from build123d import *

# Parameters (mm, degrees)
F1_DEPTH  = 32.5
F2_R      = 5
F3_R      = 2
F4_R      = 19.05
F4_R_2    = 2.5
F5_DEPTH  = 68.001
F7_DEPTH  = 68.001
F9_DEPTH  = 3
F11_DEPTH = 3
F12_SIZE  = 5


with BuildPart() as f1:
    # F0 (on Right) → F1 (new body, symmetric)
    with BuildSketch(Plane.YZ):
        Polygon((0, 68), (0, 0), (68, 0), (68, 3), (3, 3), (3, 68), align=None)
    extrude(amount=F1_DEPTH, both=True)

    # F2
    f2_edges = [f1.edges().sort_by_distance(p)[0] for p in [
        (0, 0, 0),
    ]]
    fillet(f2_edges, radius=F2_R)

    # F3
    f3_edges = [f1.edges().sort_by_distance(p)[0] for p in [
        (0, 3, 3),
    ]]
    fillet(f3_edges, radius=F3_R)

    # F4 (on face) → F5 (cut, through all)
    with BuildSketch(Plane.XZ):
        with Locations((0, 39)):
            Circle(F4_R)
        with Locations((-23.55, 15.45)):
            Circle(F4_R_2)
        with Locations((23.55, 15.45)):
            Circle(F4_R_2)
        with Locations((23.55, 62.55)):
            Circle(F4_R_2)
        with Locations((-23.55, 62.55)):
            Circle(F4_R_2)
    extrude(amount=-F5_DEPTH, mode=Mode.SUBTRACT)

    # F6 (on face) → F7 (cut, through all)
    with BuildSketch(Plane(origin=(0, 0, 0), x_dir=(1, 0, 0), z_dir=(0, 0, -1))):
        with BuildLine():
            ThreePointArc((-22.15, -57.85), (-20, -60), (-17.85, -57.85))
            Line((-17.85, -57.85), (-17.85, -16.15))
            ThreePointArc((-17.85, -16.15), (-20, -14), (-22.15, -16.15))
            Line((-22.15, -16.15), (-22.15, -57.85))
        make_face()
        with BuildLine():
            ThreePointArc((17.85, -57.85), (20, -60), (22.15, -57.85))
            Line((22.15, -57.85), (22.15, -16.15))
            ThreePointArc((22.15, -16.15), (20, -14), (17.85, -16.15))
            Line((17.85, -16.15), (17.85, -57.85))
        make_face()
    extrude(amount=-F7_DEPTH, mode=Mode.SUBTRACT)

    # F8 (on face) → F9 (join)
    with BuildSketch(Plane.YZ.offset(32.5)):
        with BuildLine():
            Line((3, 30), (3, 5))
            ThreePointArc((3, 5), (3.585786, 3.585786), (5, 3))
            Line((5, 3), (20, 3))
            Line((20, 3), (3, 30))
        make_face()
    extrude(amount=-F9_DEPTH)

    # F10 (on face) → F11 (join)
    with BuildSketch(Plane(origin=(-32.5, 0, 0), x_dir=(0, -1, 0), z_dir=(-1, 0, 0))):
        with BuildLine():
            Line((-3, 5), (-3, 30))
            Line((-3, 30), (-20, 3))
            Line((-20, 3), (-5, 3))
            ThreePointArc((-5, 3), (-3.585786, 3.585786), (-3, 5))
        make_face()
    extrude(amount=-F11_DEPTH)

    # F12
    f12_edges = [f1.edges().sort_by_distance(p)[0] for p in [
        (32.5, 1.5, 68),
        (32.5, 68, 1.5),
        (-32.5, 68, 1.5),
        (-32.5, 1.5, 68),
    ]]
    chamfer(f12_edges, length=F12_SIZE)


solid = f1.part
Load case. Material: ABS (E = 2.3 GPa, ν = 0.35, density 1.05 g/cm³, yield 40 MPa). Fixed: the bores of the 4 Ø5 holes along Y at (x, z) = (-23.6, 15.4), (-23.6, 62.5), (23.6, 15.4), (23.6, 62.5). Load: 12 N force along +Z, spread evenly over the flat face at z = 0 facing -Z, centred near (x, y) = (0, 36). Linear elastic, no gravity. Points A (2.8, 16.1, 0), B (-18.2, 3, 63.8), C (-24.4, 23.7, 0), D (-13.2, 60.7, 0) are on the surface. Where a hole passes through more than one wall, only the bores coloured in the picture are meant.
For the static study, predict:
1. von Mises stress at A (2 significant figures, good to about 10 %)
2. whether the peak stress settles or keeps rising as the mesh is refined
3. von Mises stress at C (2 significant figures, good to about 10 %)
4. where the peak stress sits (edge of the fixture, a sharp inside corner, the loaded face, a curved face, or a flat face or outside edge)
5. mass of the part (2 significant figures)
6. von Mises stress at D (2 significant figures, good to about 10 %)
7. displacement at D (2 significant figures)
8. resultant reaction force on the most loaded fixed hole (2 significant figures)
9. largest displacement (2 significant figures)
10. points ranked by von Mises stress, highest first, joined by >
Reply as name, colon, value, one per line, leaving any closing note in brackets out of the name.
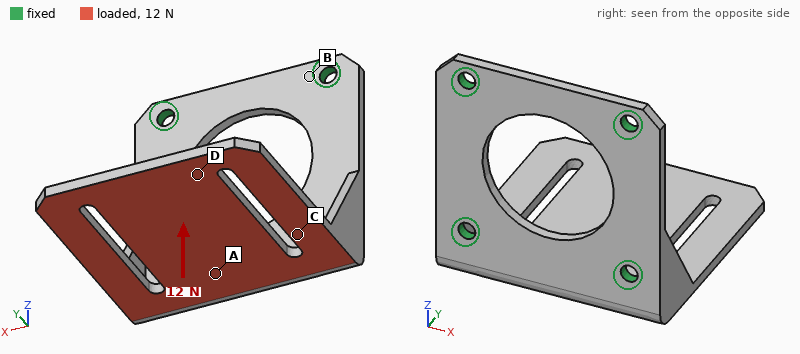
von Mises stress at A: 1.6 MPa
whether the peak stress settles or keeps rising as the mesh is refined: keeps rising
von Mises stress at C: 3.3 MPa
where the peak stress sits: edge of the fixture
mass of the part: 23 g
von Mises stress at D: 0.80 MPa
displacement at D: 1.1 mm
resultant reaction force on the most loaded fixed hole: 6.6 N
largest displacement: 1.3 mm
points ranked by von Mises stress, highest first, joined by >: C > A > D > B
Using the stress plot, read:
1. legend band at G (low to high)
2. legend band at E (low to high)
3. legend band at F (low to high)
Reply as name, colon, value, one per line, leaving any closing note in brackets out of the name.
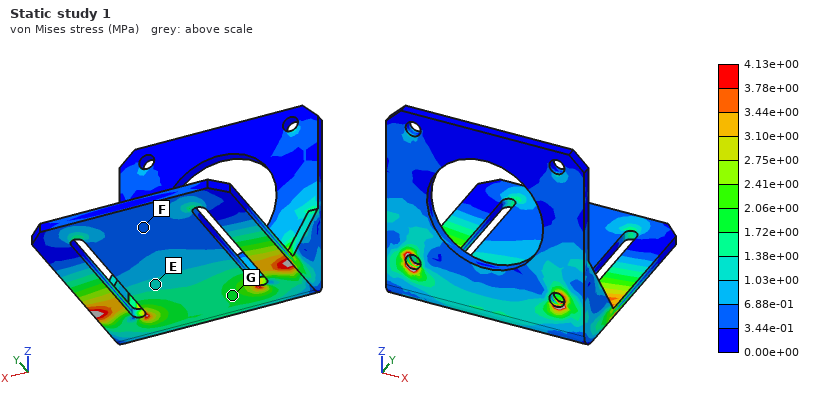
legend band at G: 1.72e+00 to 2.06e+00 MPa
legend band at E: 1.03e+00 to 1.38e+00 MPa
legend band at F: 3.44e-01 to 6.88e-01 MPa
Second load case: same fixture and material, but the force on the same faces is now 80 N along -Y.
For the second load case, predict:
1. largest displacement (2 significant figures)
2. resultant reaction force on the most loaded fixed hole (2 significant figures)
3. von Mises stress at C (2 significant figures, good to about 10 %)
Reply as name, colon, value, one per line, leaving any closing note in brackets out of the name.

largest displacement: 1.2 mm
resultant reaction force on the most loaded fixed hole: 44 N
von Mises stress at C: 1.7 MPa
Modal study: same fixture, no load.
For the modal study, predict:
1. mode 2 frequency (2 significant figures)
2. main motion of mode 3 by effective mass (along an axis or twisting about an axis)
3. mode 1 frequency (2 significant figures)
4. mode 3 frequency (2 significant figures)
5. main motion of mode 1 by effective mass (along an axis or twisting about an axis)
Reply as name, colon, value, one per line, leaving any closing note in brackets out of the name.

mode 2 frequency: 450 Hz
main motion of mode 3 by effective mass: along X
mode 1 frequency: 180 Hz
mode 3 frequency: 730 Hz
main motion of mode 1 by effective mass: along Z
